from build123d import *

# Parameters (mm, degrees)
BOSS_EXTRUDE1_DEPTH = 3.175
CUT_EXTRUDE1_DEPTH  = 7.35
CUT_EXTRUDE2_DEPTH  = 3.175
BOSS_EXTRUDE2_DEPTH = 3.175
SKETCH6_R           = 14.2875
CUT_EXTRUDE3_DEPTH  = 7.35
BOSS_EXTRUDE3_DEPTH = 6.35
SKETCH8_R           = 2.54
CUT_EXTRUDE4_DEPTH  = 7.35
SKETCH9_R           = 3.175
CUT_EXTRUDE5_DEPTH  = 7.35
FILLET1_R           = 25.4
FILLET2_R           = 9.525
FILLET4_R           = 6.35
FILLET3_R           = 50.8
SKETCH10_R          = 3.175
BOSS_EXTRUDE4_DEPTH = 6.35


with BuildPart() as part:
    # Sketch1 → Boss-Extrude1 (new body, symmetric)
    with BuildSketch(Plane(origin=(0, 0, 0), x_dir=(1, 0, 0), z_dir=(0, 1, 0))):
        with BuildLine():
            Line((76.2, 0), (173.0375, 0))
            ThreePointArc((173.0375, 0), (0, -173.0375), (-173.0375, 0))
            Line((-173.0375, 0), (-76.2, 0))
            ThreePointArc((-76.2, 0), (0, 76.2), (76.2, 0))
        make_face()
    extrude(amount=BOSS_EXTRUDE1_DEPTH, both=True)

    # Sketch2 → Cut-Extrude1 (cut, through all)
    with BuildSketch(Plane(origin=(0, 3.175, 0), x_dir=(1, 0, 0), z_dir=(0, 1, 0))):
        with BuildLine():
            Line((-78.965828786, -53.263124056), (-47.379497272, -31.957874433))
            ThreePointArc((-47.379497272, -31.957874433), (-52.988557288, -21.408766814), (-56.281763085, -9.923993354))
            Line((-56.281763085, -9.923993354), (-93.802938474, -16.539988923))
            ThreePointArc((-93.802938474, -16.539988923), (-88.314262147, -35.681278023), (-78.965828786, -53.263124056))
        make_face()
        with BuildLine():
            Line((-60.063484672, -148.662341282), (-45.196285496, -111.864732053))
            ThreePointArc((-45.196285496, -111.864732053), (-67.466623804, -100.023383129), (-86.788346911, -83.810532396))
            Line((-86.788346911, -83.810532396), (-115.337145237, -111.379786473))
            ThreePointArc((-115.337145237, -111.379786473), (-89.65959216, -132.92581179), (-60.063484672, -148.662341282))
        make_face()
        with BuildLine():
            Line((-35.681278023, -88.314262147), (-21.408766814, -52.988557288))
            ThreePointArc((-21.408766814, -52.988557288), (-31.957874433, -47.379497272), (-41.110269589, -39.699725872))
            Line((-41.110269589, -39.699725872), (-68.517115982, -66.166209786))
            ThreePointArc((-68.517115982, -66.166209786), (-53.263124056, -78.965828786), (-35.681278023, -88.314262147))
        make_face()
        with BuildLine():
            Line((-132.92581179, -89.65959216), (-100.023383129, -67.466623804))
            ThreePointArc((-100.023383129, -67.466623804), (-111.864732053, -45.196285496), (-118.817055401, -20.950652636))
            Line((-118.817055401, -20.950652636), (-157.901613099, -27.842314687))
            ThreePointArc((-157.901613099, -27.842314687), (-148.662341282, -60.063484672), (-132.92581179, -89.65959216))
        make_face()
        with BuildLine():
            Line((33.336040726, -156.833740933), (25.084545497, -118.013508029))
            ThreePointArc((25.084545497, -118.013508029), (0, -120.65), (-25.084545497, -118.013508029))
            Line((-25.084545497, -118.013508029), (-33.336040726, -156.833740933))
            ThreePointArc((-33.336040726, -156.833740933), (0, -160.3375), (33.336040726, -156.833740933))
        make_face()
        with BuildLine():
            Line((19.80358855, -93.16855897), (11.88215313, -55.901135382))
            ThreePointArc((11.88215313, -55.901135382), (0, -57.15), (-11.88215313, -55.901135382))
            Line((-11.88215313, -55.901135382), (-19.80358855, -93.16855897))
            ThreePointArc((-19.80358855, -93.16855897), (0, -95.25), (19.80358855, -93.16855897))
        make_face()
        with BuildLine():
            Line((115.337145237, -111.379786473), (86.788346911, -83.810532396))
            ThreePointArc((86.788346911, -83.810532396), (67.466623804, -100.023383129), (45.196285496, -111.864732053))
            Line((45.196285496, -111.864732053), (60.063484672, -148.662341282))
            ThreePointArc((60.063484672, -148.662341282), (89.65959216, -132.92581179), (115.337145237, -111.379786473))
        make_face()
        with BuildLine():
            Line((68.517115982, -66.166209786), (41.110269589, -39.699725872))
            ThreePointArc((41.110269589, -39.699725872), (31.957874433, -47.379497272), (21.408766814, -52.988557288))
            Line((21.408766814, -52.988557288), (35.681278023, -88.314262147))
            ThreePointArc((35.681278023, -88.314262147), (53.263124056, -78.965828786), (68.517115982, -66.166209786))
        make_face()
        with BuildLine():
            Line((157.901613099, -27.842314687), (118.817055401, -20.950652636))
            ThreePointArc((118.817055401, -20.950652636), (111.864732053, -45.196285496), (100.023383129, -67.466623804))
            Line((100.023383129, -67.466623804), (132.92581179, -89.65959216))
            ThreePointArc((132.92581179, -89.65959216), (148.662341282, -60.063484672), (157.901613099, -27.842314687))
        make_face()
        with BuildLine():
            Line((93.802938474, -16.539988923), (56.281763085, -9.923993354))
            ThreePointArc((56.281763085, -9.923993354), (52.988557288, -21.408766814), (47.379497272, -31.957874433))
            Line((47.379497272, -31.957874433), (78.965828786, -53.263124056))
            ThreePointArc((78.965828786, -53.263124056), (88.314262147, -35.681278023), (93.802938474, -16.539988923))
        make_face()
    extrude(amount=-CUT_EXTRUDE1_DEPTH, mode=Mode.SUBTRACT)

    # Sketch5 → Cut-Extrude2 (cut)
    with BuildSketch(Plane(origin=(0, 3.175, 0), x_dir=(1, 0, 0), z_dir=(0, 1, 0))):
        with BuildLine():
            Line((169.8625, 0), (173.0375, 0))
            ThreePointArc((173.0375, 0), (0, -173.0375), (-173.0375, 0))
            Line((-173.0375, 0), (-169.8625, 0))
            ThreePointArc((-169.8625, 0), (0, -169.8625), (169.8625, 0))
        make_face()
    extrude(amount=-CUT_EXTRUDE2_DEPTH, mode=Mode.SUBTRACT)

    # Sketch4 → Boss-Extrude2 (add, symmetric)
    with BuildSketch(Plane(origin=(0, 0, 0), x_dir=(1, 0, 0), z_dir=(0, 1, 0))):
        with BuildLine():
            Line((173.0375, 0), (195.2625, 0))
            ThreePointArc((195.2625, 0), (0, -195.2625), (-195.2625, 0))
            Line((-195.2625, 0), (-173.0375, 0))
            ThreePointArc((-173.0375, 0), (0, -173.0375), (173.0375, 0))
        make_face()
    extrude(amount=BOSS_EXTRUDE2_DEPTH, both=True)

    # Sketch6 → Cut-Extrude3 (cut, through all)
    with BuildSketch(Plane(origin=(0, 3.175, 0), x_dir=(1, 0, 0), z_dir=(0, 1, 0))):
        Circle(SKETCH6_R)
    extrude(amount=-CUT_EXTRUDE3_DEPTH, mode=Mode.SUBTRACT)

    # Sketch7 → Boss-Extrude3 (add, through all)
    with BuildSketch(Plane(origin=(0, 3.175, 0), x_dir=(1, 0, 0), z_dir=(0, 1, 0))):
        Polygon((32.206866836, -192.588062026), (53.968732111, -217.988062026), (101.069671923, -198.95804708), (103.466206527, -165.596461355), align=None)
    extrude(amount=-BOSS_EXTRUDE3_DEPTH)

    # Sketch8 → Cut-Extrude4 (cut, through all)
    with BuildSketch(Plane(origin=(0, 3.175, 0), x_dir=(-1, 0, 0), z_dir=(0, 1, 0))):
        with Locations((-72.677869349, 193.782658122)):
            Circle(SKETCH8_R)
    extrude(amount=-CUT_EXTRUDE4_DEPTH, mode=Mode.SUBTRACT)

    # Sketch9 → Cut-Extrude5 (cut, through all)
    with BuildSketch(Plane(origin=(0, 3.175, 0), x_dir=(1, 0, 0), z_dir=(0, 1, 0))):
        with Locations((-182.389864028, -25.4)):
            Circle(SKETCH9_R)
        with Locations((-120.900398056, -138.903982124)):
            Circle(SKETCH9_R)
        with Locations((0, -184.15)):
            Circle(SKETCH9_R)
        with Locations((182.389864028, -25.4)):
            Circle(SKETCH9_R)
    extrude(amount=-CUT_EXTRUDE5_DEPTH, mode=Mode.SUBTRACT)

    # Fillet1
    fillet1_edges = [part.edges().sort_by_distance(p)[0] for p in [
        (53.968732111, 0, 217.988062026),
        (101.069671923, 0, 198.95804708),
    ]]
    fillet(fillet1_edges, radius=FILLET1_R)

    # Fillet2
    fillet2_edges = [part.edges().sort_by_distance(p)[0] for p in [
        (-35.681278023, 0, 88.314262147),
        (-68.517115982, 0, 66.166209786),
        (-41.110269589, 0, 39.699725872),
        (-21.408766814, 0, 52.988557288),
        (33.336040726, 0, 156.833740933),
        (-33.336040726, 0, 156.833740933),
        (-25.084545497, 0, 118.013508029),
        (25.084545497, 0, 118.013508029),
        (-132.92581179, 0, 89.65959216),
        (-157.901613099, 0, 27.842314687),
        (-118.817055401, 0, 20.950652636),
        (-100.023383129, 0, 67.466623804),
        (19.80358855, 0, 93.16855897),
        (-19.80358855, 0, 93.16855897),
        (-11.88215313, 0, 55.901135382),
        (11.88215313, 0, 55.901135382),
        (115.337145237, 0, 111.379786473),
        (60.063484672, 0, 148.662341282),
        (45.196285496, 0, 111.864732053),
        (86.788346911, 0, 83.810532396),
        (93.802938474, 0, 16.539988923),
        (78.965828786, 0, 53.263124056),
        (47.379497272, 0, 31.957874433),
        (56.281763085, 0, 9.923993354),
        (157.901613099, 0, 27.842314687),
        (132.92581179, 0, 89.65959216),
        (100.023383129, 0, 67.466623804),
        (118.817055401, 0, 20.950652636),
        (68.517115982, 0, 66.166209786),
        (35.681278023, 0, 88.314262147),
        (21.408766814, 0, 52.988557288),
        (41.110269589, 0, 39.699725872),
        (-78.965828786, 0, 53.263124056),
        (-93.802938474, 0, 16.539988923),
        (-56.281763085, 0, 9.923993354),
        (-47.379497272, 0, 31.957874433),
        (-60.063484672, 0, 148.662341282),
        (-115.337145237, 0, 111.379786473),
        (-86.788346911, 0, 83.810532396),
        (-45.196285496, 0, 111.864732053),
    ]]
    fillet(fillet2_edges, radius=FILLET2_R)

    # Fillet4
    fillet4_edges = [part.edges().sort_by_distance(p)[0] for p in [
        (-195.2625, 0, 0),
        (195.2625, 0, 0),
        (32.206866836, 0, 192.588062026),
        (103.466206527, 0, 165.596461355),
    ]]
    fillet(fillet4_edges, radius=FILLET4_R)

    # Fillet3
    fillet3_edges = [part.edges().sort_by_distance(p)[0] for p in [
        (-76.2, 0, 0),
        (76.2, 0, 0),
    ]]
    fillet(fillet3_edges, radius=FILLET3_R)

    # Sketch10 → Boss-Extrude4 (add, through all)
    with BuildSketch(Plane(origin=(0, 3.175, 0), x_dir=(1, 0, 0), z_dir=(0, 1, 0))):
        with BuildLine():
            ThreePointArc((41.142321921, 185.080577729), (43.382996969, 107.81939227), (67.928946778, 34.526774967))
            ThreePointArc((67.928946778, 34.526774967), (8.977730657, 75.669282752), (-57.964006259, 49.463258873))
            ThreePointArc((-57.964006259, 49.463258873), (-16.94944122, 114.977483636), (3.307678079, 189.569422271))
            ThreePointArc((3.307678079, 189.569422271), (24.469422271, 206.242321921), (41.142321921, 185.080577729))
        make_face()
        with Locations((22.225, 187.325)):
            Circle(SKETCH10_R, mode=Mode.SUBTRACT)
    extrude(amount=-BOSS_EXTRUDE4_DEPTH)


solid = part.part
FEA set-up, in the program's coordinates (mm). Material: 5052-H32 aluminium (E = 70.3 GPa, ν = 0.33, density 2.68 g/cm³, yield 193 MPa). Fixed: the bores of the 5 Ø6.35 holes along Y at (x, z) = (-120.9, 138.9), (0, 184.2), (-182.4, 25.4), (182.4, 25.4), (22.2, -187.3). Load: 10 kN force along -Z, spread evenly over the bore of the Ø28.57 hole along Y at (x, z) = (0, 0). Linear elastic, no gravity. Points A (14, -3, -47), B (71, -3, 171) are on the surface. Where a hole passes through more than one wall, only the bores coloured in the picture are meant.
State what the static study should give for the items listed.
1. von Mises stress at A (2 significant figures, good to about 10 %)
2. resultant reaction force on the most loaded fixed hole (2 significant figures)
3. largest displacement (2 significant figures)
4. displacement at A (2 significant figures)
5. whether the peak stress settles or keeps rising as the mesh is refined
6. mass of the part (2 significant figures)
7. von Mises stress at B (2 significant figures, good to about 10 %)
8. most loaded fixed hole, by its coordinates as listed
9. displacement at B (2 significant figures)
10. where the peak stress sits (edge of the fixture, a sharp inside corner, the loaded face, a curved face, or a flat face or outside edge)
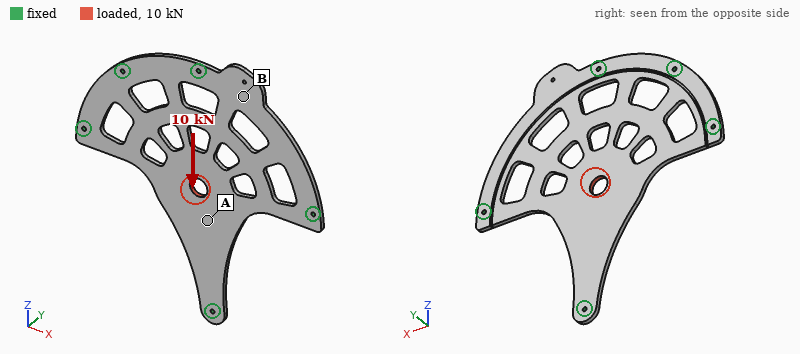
14 MPa
5.1 kN
49 µm
38 µm
keeps rising
1.0 kg
5.0 MPa
(22.2, -187.3)
19 µm
edge of the fixture
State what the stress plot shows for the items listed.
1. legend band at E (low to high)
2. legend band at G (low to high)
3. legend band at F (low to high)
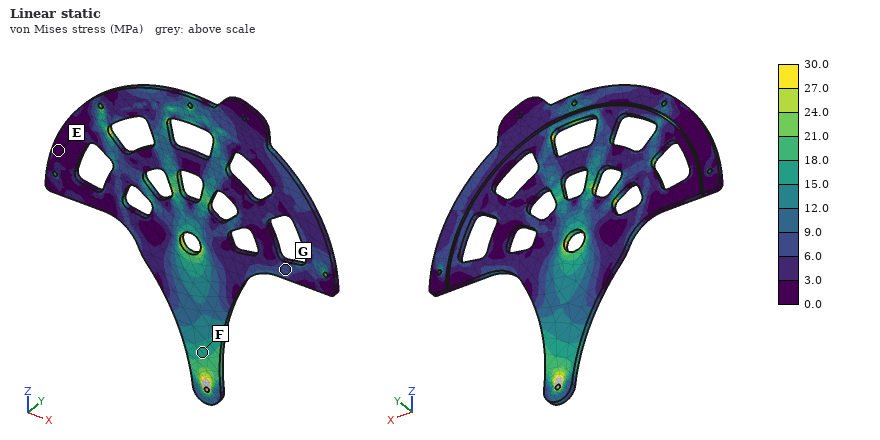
0.0 to 3.0 MPa
6.0 to 9.0 MPa
15.0 to 18.0 MPa
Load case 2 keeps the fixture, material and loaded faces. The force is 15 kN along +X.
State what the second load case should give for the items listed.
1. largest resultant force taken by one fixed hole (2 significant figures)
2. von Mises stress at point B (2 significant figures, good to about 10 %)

5.5 kN
8.0 MPa
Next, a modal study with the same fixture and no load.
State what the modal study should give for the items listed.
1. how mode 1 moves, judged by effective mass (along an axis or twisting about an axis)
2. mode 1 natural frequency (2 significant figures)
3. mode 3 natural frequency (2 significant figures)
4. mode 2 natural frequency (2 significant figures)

along Y
260 Hz
600 Hz
440 Hz
